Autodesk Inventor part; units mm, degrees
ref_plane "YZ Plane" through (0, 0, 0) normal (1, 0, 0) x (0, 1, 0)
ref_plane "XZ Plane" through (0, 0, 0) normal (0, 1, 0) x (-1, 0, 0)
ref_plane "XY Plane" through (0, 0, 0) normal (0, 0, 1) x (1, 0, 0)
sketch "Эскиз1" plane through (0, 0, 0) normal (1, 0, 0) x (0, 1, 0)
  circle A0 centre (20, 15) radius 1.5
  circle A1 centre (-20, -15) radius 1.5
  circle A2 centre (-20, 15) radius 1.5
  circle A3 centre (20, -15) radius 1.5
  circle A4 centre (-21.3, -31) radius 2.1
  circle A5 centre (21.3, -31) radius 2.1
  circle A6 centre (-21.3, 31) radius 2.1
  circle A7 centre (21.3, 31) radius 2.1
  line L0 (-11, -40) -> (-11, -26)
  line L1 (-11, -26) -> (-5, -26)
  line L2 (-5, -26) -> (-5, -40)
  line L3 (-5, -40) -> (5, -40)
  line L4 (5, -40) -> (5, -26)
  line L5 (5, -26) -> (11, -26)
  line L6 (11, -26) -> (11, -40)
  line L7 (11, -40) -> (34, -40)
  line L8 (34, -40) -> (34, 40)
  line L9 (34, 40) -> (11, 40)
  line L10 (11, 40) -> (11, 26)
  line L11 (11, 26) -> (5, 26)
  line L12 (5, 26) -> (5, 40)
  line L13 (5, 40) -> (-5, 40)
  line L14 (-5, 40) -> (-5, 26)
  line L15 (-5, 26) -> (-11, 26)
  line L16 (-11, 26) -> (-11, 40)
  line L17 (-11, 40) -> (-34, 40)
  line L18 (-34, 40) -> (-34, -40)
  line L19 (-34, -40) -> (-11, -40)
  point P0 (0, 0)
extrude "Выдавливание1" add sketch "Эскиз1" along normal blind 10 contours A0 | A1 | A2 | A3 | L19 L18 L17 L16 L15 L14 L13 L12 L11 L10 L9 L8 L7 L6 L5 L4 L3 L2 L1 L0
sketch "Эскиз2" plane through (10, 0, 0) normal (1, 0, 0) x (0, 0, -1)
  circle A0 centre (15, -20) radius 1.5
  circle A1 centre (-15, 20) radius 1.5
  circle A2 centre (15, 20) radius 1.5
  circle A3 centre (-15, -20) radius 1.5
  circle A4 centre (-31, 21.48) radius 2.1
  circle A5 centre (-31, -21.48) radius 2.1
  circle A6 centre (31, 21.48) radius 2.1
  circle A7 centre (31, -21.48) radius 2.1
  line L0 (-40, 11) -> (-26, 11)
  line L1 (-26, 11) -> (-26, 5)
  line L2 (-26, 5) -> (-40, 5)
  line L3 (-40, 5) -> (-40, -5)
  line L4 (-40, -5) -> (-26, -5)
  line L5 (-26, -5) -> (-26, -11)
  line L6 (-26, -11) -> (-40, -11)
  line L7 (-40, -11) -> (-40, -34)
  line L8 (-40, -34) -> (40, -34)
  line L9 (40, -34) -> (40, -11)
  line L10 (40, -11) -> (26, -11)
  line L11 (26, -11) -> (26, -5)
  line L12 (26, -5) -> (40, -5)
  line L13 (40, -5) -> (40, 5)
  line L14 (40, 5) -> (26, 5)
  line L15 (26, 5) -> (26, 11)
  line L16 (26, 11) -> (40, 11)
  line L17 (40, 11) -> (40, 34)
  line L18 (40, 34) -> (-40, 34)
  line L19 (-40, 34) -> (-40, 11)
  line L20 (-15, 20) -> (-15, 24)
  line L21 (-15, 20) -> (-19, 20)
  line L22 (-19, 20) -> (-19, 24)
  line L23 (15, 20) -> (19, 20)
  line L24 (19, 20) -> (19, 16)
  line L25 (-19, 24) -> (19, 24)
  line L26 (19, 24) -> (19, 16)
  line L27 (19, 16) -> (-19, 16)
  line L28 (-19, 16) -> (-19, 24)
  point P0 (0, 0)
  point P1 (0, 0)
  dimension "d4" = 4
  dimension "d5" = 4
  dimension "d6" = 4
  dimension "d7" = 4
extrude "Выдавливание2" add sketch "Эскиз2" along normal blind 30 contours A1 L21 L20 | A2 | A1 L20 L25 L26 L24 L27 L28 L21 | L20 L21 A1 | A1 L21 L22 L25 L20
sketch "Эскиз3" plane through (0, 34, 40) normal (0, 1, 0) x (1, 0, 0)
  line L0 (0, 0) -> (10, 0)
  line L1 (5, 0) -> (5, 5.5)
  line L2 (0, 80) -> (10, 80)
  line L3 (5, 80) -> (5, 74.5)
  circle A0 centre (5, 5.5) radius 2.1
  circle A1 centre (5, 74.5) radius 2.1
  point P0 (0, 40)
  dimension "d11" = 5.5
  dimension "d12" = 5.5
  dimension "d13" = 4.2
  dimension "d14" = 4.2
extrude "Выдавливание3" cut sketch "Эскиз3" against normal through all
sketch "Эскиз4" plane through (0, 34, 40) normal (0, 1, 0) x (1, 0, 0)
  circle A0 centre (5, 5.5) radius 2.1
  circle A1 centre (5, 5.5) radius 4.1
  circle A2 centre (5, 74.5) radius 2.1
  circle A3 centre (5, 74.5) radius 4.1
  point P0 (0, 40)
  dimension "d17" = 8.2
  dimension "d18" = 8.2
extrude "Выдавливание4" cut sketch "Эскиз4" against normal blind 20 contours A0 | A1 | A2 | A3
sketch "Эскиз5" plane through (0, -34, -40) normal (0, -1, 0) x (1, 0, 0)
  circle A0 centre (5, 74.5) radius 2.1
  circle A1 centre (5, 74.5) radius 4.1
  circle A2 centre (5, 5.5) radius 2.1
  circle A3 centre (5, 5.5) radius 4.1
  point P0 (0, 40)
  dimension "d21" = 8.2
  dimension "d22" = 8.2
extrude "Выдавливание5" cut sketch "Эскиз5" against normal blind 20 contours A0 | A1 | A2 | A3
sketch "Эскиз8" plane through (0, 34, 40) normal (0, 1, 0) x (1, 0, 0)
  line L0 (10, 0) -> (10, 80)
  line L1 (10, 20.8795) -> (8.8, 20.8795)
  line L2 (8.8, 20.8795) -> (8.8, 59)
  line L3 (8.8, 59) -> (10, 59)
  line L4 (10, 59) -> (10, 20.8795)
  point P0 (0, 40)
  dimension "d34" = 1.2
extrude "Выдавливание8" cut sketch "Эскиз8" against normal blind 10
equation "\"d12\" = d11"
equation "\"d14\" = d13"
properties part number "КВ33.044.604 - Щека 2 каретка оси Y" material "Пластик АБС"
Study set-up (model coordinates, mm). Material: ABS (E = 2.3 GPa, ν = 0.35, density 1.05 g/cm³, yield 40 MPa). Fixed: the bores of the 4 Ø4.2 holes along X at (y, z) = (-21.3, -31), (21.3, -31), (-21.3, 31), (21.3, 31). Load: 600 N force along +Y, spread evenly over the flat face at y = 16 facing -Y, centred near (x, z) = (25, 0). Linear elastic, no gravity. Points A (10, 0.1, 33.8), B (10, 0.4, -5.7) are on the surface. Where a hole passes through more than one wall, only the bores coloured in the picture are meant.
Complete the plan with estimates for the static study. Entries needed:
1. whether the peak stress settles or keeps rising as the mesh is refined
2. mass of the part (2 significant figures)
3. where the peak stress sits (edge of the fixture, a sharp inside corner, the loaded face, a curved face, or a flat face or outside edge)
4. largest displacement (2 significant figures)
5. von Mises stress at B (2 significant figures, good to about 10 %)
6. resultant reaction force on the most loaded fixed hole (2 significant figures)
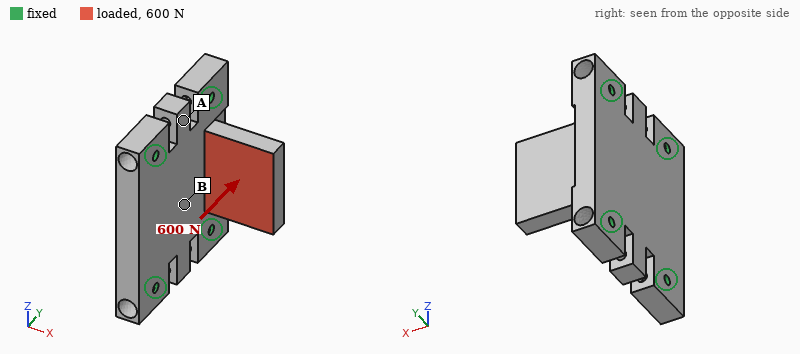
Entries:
keeps rising
57 g
a sharp inside corner
1.1 mm
4.3 MPa
190 N
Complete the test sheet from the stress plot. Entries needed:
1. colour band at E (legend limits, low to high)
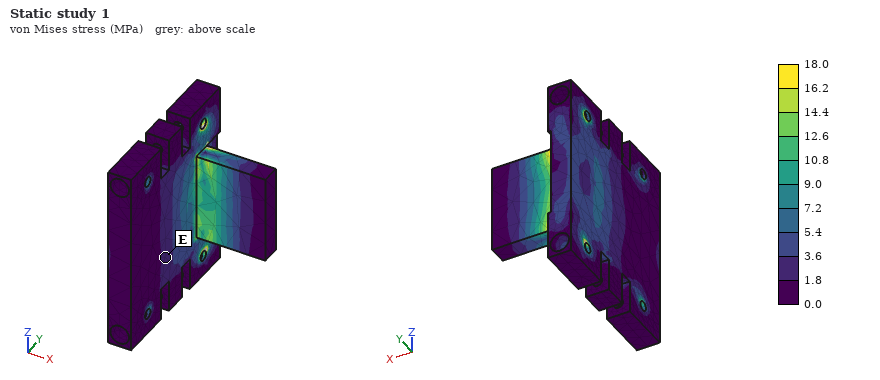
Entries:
1.8 to 3.6 MPa
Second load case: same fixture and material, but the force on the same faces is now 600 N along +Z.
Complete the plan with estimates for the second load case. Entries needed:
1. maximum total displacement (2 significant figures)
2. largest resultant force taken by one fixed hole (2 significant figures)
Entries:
0.22 mm
340 N
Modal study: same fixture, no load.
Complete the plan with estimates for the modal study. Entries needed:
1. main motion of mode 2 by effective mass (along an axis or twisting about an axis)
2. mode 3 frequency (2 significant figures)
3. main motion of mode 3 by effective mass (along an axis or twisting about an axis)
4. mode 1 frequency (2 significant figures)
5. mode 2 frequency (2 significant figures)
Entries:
along X
3300 Hz
twisting about Z
1400 Hz
2600 Hz
